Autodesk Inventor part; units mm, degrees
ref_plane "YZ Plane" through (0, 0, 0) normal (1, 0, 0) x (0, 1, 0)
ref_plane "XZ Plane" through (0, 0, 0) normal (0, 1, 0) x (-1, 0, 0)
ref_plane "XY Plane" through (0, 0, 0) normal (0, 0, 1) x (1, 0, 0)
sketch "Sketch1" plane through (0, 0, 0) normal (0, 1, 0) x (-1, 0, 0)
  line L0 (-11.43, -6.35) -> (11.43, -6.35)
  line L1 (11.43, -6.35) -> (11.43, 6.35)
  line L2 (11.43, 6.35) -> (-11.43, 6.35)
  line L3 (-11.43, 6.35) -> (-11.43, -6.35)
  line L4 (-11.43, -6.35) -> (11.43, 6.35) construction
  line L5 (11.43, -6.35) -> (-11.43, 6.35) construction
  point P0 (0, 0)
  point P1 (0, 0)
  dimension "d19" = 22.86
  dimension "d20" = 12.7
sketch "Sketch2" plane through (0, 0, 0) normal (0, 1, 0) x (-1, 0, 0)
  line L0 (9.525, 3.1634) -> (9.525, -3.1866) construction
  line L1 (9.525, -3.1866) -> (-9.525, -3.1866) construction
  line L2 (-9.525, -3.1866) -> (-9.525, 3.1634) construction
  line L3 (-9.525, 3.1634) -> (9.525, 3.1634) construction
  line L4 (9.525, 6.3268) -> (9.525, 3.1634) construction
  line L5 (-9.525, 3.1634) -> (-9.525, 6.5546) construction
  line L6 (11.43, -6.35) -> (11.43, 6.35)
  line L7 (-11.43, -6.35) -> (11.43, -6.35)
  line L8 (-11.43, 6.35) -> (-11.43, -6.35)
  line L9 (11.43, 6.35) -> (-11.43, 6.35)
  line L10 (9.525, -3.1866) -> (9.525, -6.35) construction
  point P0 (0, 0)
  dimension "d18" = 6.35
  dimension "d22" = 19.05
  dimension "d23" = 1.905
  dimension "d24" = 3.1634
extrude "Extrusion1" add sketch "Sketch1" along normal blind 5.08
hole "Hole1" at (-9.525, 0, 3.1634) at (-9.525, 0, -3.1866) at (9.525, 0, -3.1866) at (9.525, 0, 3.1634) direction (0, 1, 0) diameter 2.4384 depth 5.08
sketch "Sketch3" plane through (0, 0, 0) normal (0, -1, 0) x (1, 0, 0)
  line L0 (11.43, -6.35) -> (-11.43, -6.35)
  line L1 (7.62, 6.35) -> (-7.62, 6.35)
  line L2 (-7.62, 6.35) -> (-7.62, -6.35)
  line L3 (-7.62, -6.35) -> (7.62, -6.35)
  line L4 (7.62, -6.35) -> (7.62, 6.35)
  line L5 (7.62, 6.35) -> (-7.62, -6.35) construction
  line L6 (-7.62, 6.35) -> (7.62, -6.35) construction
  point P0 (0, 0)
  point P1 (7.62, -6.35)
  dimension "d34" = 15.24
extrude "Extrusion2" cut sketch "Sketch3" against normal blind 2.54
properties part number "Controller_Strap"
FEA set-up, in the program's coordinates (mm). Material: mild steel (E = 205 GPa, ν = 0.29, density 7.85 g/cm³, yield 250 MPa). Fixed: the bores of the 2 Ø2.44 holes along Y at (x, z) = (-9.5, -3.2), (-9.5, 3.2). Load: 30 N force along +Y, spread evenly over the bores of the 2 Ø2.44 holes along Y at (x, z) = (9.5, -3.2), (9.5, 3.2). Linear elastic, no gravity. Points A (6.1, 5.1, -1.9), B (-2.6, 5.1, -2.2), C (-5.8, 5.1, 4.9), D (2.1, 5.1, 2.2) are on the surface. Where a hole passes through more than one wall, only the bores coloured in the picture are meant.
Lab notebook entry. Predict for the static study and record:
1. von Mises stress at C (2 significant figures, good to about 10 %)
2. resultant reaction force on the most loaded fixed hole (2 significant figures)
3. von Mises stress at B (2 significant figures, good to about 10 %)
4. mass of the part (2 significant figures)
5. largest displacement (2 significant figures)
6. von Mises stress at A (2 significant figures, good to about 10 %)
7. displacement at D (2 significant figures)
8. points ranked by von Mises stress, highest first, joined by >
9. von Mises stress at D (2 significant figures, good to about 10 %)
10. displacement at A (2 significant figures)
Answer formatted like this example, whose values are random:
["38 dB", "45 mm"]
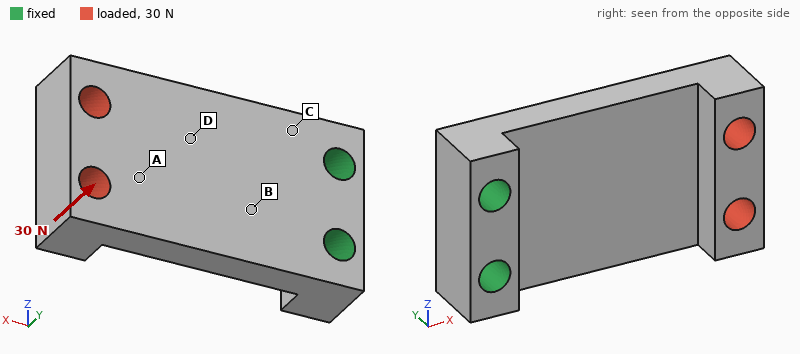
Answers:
["32 MPa", "15 N", "25 MPa", "7.0 g", "20 µm", "7.6 MPa", "7.0 µm", "C > B > D > A", "16 MPa", "12 µm"]
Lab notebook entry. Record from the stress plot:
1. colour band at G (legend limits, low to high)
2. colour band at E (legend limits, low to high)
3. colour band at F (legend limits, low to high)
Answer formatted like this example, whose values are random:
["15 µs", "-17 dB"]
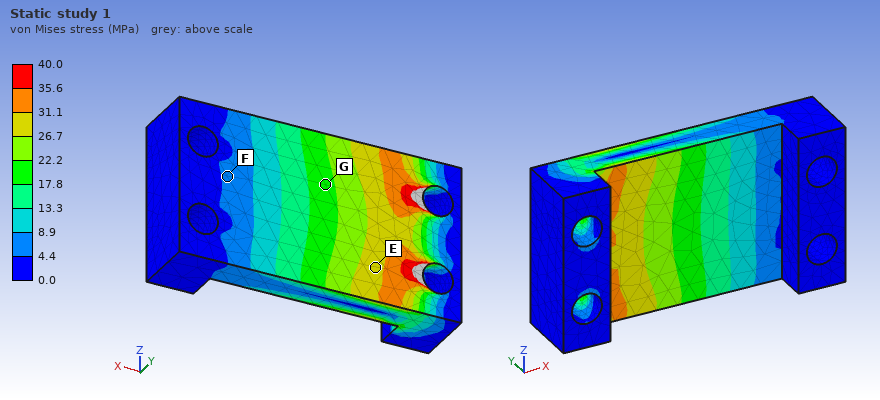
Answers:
["17.8 to 22.2 MPa", "26.7 to 31.1 MPa", "4.4 to 8.9 MPa"]
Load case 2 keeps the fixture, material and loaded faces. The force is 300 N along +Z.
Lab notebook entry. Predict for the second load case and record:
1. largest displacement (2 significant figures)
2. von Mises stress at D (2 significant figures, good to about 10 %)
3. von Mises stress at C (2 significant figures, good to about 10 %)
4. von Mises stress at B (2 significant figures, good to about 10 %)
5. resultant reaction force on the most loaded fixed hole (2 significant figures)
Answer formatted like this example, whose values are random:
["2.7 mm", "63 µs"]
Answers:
["18 µm", "11 MPa", "62 MPa", "21 MPa", "690 N"]
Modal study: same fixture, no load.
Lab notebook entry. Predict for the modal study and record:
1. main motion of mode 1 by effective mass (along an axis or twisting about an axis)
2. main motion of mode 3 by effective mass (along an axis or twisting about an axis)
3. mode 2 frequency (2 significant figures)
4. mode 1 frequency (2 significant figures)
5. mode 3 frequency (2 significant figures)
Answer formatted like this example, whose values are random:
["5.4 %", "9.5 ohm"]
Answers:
["along Y", "along Z", "14 kHz", "4500 Hz", "18 kHz"]
